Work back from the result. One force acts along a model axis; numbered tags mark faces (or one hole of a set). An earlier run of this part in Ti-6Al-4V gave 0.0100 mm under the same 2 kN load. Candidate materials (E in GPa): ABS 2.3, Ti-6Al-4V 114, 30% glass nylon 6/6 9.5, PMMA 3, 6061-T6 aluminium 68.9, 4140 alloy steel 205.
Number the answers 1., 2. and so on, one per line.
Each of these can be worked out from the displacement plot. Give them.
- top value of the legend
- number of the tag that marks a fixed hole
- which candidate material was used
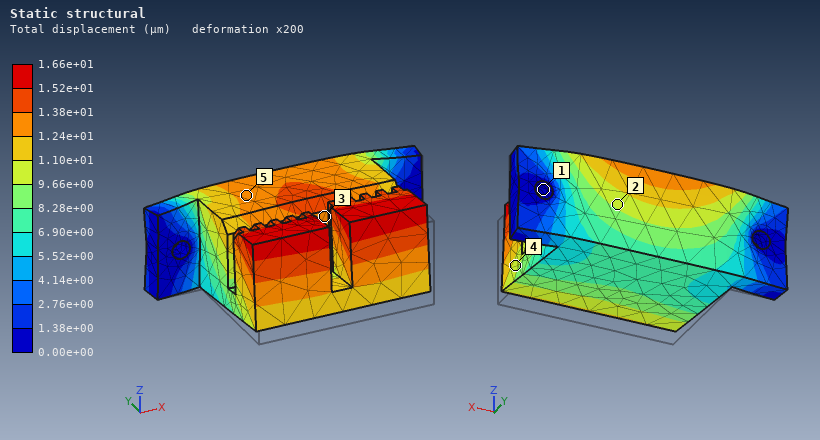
1. 1.66e+01 µm
2. 1
3. 6061-T6 aluminium
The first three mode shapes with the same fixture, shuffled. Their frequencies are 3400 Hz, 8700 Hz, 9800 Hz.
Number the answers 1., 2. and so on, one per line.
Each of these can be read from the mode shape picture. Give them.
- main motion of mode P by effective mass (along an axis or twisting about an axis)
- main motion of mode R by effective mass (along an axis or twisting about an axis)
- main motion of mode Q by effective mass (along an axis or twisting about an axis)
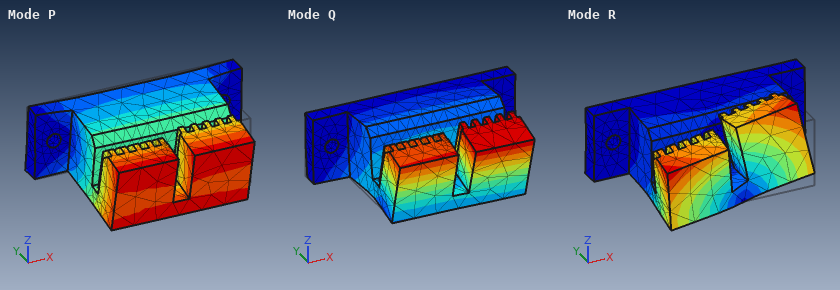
1. along Z
2. along X
3. along Y
